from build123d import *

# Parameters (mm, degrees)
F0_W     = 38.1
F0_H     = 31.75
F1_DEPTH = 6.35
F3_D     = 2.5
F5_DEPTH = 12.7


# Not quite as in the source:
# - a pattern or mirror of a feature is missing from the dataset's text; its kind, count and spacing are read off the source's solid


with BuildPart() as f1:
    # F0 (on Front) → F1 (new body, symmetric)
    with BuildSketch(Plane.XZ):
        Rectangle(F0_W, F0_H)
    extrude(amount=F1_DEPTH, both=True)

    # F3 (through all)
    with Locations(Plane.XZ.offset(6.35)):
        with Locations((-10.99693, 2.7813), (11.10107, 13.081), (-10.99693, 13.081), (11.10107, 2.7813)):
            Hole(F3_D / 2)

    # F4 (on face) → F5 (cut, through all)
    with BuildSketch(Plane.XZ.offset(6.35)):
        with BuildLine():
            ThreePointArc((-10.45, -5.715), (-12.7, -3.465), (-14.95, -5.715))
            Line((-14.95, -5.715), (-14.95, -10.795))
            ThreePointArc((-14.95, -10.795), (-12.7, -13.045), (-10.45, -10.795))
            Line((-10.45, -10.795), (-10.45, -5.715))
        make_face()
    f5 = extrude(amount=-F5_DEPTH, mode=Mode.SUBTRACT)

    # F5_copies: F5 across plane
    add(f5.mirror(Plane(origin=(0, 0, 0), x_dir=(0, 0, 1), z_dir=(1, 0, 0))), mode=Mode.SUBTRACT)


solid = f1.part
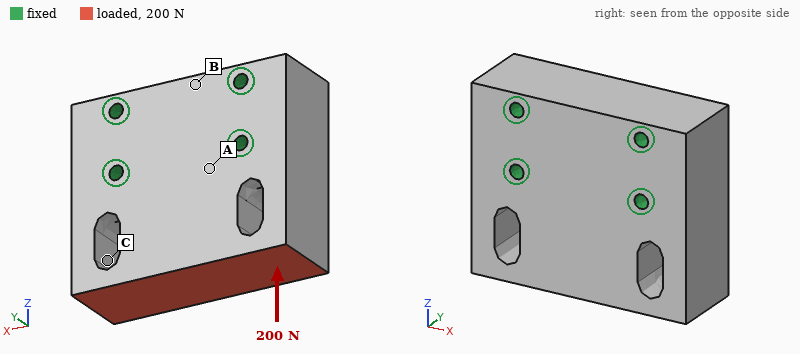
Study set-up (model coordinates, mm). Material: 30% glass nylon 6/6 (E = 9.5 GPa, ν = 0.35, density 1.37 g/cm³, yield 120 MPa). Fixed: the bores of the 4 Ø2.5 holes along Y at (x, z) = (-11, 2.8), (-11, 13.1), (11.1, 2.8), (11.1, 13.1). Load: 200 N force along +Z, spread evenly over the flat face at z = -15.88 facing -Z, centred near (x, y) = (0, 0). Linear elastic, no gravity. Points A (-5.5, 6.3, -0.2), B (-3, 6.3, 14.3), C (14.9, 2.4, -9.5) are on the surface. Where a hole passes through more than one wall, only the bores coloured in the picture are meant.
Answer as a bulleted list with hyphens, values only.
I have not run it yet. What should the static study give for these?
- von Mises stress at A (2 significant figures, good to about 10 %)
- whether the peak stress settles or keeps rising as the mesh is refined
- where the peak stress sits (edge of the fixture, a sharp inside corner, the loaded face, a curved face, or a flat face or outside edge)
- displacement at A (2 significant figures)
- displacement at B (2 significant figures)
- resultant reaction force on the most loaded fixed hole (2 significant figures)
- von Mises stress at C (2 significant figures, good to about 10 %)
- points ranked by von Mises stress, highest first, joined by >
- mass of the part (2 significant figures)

- 0.36 MPa
- keeps rising
- edge of the fixture
- 0.45 µm
- 0.29 µm
- 75 N
- 0.97 MPa
- C > A > B
- 19 g
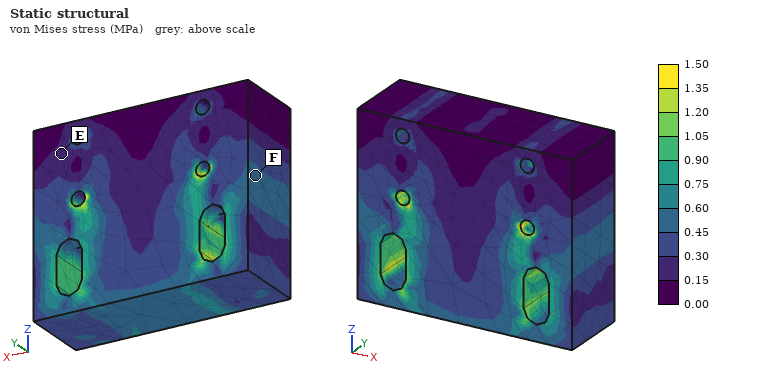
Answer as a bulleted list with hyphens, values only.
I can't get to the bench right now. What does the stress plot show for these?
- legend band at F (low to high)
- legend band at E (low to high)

- 0.45 to 0.60 MPa
- 0.15 to 0.30 MPa
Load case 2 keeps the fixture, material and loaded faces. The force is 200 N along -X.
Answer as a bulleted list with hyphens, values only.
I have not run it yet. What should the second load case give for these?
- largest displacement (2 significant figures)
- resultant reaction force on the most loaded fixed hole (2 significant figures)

- 6.3 µm
- 160 N
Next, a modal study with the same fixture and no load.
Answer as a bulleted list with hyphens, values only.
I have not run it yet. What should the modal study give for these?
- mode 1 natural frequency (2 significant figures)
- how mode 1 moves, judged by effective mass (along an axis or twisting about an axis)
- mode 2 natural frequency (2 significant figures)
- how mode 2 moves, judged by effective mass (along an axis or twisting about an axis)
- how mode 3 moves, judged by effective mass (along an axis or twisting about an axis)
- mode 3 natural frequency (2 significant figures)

- 9800 Hz
- along Y
- 14 kHz
- twisting about Z
- along X
- 15 kHz
